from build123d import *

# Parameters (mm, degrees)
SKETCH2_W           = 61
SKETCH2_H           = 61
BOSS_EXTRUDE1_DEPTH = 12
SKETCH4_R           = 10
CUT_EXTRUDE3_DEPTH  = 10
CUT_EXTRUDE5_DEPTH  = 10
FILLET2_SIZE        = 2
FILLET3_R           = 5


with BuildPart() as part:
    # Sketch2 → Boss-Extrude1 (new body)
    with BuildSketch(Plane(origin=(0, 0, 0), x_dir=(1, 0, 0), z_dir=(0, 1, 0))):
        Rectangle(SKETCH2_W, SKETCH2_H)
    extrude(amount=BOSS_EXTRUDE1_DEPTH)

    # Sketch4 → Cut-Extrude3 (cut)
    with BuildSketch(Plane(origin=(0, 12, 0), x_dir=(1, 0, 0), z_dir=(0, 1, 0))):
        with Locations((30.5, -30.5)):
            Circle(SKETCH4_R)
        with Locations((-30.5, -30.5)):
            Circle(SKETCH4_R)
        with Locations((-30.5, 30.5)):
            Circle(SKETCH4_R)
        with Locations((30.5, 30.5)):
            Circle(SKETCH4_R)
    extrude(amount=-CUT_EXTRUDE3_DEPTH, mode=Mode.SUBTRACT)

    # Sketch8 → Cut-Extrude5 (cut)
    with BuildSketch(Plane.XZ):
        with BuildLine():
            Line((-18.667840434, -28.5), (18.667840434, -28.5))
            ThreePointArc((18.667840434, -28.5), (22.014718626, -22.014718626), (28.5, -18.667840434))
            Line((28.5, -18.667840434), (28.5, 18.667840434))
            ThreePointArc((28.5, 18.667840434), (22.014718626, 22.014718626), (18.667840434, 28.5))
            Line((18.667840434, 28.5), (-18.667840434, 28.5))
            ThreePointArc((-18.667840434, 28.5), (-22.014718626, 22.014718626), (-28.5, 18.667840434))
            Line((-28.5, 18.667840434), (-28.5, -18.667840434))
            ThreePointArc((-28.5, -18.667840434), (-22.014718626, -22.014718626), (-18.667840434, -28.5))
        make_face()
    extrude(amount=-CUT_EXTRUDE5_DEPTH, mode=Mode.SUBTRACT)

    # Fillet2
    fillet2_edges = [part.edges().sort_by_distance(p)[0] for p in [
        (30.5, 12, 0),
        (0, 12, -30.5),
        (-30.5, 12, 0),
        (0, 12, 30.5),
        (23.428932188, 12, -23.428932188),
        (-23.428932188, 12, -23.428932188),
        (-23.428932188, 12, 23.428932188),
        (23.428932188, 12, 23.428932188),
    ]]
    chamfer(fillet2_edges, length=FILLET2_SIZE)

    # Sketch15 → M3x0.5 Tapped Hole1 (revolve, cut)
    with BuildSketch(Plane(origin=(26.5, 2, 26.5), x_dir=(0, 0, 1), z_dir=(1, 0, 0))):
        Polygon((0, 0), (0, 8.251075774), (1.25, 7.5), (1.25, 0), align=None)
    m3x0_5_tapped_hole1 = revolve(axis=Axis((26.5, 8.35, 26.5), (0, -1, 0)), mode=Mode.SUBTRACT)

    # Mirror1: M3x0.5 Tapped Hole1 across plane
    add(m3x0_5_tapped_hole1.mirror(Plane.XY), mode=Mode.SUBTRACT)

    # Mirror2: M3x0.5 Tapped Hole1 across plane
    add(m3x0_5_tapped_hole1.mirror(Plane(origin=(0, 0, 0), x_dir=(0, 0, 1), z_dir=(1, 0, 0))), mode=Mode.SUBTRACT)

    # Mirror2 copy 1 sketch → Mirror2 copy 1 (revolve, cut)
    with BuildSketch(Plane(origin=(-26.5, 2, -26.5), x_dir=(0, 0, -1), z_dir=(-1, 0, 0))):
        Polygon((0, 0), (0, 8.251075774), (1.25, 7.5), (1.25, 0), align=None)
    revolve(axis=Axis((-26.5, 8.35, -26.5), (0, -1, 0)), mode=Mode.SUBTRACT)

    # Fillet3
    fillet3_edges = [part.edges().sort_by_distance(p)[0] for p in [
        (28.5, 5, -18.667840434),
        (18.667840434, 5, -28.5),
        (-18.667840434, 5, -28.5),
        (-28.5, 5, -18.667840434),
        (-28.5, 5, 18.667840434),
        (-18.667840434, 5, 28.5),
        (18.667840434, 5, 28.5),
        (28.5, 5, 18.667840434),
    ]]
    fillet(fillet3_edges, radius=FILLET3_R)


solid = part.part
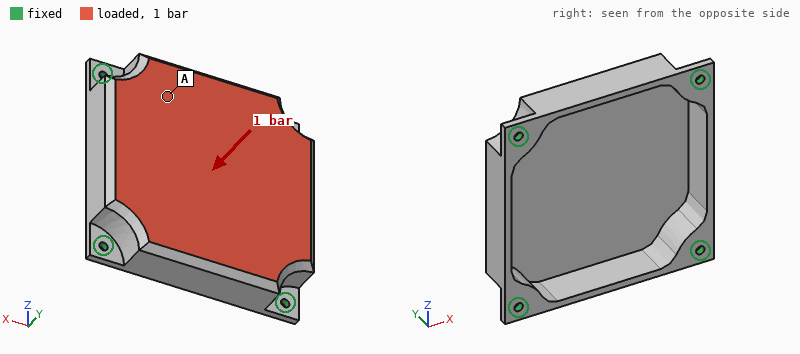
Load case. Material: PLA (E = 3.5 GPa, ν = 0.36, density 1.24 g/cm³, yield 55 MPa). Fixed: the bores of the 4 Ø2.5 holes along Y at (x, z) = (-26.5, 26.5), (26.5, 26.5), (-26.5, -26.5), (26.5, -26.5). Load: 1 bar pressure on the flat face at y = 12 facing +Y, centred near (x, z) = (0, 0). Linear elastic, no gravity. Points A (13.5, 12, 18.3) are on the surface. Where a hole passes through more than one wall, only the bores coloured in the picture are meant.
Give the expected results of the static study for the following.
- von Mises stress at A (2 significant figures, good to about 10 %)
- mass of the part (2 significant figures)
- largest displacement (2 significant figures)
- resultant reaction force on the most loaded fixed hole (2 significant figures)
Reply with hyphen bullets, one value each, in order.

- 6.0 MPa
- 14 g
- 0.89 mm
- 94 N
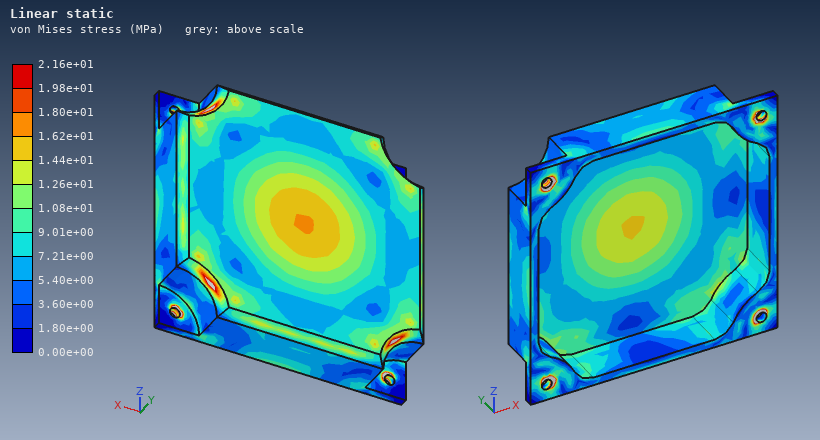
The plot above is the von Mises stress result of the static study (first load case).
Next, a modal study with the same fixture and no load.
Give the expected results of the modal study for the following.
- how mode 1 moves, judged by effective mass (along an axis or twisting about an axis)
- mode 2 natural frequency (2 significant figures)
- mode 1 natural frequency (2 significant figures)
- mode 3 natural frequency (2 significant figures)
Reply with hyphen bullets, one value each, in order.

- along Y
- 2600 Hz
- 1300 Hz
- 2600 Hz
